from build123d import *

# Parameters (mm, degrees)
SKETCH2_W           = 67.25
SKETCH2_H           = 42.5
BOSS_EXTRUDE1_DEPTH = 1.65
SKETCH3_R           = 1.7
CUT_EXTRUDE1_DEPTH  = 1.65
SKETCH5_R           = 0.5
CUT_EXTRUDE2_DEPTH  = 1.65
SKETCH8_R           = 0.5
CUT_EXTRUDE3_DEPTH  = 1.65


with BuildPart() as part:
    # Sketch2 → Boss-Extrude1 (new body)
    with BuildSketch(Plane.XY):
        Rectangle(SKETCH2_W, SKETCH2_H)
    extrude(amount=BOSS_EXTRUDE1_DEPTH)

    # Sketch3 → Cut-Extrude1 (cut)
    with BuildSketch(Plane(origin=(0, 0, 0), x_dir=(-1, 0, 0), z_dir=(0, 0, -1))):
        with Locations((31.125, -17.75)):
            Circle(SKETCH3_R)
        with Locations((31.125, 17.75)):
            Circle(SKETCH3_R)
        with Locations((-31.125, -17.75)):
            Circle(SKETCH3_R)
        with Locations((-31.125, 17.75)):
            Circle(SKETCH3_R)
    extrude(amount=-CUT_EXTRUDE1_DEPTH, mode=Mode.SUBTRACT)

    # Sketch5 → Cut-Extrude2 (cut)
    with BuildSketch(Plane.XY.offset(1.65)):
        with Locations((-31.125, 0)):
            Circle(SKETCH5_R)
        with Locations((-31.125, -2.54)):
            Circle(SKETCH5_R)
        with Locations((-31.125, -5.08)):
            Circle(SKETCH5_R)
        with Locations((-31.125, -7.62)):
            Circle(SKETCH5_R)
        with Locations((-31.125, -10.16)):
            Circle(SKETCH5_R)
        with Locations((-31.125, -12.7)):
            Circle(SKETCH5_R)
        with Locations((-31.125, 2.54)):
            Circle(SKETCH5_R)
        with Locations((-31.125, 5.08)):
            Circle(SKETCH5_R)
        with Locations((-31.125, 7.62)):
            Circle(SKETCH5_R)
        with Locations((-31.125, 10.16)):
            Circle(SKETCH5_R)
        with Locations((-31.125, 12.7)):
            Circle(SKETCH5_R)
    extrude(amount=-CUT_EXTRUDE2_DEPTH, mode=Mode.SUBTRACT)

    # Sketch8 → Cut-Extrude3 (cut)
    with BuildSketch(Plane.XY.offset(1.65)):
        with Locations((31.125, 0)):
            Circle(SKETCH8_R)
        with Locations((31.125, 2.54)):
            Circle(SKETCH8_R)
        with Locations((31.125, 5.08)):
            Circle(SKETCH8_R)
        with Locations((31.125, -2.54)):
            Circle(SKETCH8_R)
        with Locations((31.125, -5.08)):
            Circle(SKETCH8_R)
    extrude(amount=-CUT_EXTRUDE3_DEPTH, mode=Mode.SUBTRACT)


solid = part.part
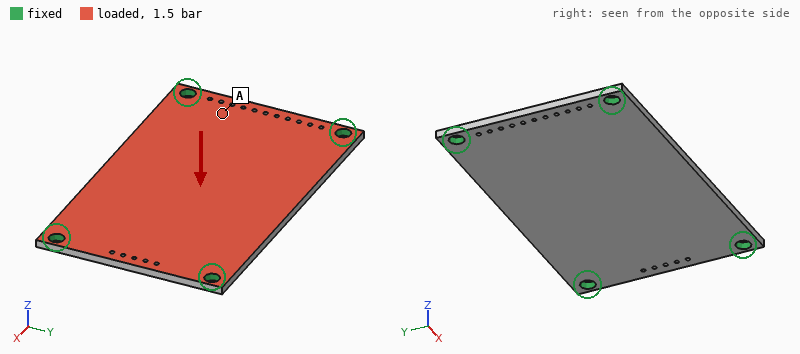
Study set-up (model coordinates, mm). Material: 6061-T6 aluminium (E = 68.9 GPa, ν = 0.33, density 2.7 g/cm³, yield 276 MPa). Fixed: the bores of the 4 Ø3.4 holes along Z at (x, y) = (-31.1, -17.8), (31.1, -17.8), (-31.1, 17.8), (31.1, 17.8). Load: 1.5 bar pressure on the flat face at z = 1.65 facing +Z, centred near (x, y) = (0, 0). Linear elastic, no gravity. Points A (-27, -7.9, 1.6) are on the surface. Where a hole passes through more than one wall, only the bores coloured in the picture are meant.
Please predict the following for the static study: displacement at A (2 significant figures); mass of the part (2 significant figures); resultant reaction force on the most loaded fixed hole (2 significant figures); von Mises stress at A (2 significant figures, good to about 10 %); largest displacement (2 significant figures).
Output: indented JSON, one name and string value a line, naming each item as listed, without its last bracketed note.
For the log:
{
  "displacement at A": "0.051 mm",
  "mass of the part": "13 g",
  "resultant reaction force on the most loaded fixed hole": "110 N",
  "von Mises stress at A": "32 MPa",
  "largest displacement": "0.28 mm"
}
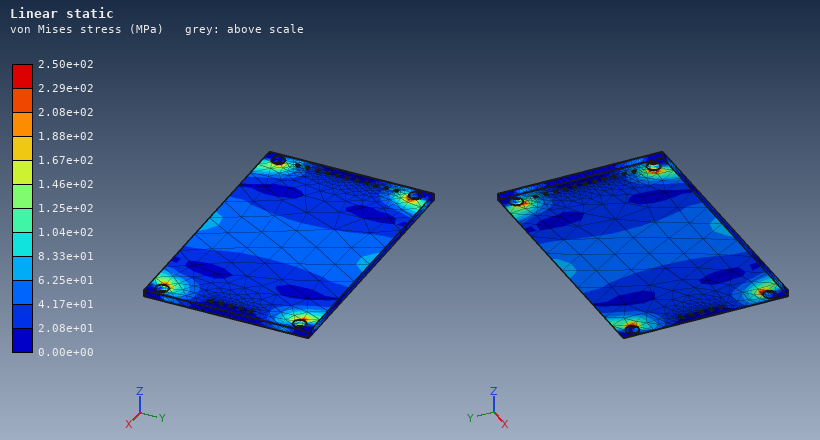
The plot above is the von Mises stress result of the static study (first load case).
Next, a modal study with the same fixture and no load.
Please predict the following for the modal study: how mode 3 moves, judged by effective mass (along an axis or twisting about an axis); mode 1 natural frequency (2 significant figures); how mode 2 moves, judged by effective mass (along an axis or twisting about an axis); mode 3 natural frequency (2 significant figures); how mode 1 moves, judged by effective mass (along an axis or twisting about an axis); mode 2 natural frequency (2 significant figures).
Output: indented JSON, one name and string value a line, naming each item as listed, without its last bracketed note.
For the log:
{
  "how mode 3 moves, judged by effective mass": "twisting about Y",
  "mode 1 natural frequency": "2000 Hz",
  "how mode 2 moves, judged by effective mass": "twisting about X",
  "mode 3 natural frequency": "5200 Hz",
  "how mode 1 moves, judged by effective mass": "along Z",
  "mode 2 natural frequency": "3200 Hz"
}
